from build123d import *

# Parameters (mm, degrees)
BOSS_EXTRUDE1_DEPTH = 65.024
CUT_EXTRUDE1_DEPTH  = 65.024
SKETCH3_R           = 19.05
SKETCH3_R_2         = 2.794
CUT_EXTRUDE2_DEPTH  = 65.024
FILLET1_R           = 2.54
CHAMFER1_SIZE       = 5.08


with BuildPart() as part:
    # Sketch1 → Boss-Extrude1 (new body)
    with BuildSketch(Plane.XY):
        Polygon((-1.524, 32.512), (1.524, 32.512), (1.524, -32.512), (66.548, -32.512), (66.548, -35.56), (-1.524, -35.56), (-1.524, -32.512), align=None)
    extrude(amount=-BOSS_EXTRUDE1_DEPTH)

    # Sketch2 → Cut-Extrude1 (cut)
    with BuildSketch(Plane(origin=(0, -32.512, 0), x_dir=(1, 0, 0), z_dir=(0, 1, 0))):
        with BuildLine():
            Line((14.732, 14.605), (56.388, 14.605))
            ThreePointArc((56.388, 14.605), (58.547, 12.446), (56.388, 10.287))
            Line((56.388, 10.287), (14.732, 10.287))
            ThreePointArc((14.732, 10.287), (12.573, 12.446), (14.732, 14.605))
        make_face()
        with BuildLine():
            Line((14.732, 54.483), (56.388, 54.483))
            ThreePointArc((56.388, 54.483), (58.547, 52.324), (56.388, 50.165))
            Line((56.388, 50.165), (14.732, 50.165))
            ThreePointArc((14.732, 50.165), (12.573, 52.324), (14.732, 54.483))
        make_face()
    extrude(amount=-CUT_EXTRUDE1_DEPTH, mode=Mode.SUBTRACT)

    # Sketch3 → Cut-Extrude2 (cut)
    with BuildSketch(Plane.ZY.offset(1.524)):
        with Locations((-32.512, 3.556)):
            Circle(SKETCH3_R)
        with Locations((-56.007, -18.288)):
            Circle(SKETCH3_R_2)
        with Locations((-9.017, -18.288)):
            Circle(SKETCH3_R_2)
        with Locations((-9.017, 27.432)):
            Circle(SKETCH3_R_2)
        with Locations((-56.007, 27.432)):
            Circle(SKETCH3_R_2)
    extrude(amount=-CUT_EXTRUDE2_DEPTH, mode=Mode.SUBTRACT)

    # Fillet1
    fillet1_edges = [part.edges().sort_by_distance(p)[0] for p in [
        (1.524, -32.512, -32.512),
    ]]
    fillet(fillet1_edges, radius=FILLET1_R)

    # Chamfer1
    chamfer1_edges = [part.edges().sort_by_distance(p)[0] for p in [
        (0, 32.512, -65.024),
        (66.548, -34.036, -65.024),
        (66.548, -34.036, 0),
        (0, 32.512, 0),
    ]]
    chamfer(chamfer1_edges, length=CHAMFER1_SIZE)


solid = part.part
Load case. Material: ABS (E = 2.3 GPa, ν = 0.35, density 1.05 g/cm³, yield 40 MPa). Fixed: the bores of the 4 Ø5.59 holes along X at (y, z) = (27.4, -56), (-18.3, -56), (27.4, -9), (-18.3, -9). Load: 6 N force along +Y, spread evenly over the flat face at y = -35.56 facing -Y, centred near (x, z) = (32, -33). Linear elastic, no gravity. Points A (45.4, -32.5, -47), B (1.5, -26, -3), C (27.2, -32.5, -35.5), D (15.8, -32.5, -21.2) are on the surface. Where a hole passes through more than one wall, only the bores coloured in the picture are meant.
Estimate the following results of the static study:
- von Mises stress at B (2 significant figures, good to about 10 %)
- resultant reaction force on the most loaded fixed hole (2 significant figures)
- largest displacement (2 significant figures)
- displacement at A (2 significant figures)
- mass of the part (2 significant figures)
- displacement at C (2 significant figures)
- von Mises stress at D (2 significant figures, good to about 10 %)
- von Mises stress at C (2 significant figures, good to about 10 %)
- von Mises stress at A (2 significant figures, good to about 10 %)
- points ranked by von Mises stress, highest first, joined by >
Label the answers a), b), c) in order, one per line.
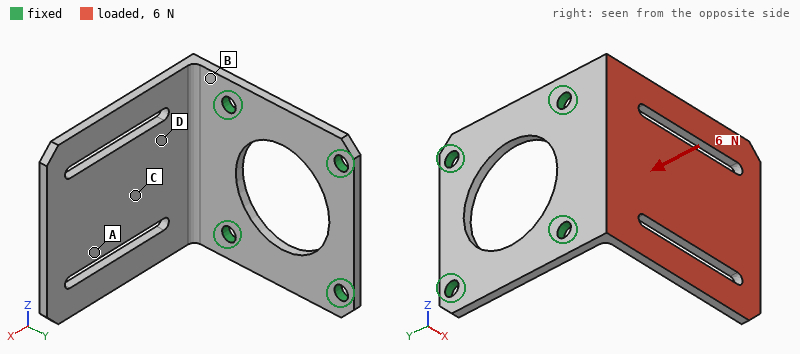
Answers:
a) 2.0 MPa
b) 3.3 N
c) 1.1 mm
d) 0.66 mm
e) 22 g
f) 0.34 mm
g) 1.2 MPa
h) 0.73 MPa
i) 0.27 MPa
j) B > D > C > A
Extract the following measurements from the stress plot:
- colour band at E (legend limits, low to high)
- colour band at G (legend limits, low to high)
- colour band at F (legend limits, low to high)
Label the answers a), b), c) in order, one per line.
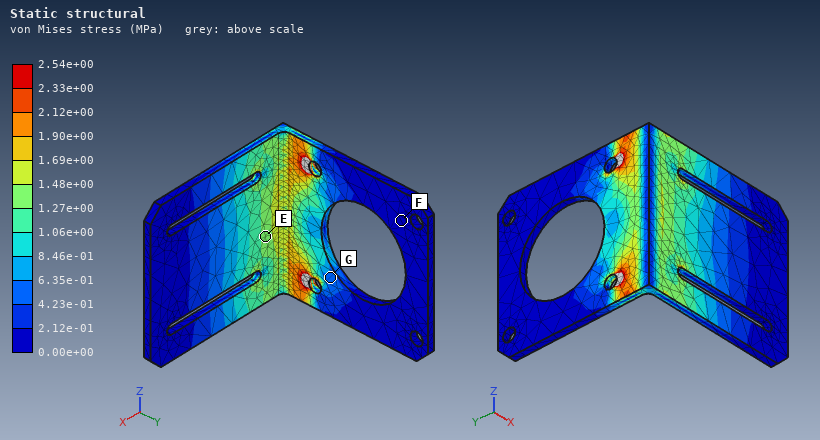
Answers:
a) 1.27e+00 to 1.48e+00 MPa
b) 4.23e-01 to 6.35e-01 MPa
c) 0.00e+00 to 2.12e-01 MPa
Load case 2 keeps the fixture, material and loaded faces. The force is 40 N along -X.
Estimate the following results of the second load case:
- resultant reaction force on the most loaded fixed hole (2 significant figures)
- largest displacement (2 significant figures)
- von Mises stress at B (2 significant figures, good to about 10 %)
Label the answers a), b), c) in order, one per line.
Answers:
a) 20 N
b) 1.3 mm
c) 4.6 MPa
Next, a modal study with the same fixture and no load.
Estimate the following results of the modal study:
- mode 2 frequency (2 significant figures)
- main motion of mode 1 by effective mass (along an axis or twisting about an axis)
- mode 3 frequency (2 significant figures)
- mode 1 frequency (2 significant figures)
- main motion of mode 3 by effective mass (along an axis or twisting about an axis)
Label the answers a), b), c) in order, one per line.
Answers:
a) 360 Hz
b) along Y
c) 560 Hz
d) 130 Hz
e) along Z
